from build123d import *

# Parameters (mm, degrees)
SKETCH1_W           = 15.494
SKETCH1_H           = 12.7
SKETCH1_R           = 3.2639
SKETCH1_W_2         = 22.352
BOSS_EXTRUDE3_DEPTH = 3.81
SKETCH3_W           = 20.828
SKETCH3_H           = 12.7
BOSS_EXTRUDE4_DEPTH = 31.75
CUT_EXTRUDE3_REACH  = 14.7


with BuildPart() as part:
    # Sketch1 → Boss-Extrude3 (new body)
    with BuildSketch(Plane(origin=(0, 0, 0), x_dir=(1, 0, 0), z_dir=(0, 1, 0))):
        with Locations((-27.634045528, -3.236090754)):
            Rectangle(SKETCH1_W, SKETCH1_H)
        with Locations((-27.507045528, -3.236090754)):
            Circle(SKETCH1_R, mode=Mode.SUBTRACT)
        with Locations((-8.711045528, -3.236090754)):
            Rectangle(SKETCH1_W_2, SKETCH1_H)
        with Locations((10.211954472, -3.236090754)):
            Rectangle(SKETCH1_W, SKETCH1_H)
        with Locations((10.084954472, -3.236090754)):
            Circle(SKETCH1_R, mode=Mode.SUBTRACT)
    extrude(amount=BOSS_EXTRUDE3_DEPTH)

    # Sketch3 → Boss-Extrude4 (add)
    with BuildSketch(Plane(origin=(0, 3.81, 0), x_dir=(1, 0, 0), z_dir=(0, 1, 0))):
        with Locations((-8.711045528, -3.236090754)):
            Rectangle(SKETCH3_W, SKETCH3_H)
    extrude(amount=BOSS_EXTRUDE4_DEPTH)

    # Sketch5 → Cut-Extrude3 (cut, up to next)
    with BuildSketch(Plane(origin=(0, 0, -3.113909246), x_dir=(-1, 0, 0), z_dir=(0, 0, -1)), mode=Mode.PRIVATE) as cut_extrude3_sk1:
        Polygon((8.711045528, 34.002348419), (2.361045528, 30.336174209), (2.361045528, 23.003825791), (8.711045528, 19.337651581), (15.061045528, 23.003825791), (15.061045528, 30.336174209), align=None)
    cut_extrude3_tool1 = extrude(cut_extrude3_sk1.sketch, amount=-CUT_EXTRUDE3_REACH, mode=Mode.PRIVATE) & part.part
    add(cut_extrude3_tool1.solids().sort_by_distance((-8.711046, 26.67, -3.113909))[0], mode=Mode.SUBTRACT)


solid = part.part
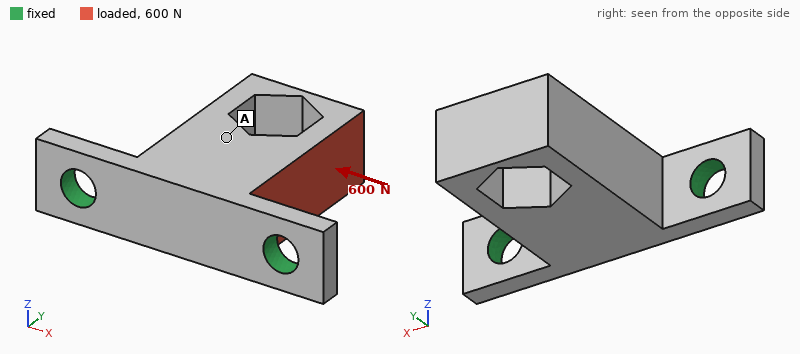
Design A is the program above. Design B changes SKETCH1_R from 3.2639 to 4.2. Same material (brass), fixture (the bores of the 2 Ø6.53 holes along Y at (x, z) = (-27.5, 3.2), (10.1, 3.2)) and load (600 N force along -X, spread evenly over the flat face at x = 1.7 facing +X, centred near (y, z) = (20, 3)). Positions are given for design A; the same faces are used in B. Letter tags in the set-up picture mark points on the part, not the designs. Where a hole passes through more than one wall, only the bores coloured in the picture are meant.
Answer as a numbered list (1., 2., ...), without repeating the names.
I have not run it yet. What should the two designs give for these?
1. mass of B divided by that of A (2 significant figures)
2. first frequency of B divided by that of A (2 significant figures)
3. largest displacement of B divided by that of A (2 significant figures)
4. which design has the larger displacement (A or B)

1. 0.98
2. 1.1
3. 0.86
4. A
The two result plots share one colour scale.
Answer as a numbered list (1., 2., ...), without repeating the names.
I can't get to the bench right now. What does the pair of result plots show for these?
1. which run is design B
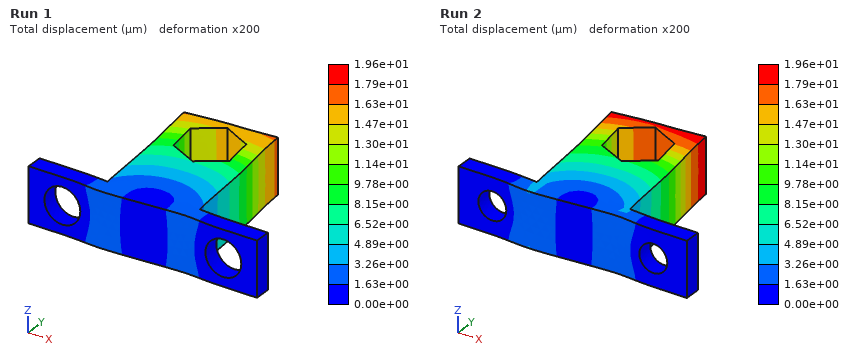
1. Run 1
